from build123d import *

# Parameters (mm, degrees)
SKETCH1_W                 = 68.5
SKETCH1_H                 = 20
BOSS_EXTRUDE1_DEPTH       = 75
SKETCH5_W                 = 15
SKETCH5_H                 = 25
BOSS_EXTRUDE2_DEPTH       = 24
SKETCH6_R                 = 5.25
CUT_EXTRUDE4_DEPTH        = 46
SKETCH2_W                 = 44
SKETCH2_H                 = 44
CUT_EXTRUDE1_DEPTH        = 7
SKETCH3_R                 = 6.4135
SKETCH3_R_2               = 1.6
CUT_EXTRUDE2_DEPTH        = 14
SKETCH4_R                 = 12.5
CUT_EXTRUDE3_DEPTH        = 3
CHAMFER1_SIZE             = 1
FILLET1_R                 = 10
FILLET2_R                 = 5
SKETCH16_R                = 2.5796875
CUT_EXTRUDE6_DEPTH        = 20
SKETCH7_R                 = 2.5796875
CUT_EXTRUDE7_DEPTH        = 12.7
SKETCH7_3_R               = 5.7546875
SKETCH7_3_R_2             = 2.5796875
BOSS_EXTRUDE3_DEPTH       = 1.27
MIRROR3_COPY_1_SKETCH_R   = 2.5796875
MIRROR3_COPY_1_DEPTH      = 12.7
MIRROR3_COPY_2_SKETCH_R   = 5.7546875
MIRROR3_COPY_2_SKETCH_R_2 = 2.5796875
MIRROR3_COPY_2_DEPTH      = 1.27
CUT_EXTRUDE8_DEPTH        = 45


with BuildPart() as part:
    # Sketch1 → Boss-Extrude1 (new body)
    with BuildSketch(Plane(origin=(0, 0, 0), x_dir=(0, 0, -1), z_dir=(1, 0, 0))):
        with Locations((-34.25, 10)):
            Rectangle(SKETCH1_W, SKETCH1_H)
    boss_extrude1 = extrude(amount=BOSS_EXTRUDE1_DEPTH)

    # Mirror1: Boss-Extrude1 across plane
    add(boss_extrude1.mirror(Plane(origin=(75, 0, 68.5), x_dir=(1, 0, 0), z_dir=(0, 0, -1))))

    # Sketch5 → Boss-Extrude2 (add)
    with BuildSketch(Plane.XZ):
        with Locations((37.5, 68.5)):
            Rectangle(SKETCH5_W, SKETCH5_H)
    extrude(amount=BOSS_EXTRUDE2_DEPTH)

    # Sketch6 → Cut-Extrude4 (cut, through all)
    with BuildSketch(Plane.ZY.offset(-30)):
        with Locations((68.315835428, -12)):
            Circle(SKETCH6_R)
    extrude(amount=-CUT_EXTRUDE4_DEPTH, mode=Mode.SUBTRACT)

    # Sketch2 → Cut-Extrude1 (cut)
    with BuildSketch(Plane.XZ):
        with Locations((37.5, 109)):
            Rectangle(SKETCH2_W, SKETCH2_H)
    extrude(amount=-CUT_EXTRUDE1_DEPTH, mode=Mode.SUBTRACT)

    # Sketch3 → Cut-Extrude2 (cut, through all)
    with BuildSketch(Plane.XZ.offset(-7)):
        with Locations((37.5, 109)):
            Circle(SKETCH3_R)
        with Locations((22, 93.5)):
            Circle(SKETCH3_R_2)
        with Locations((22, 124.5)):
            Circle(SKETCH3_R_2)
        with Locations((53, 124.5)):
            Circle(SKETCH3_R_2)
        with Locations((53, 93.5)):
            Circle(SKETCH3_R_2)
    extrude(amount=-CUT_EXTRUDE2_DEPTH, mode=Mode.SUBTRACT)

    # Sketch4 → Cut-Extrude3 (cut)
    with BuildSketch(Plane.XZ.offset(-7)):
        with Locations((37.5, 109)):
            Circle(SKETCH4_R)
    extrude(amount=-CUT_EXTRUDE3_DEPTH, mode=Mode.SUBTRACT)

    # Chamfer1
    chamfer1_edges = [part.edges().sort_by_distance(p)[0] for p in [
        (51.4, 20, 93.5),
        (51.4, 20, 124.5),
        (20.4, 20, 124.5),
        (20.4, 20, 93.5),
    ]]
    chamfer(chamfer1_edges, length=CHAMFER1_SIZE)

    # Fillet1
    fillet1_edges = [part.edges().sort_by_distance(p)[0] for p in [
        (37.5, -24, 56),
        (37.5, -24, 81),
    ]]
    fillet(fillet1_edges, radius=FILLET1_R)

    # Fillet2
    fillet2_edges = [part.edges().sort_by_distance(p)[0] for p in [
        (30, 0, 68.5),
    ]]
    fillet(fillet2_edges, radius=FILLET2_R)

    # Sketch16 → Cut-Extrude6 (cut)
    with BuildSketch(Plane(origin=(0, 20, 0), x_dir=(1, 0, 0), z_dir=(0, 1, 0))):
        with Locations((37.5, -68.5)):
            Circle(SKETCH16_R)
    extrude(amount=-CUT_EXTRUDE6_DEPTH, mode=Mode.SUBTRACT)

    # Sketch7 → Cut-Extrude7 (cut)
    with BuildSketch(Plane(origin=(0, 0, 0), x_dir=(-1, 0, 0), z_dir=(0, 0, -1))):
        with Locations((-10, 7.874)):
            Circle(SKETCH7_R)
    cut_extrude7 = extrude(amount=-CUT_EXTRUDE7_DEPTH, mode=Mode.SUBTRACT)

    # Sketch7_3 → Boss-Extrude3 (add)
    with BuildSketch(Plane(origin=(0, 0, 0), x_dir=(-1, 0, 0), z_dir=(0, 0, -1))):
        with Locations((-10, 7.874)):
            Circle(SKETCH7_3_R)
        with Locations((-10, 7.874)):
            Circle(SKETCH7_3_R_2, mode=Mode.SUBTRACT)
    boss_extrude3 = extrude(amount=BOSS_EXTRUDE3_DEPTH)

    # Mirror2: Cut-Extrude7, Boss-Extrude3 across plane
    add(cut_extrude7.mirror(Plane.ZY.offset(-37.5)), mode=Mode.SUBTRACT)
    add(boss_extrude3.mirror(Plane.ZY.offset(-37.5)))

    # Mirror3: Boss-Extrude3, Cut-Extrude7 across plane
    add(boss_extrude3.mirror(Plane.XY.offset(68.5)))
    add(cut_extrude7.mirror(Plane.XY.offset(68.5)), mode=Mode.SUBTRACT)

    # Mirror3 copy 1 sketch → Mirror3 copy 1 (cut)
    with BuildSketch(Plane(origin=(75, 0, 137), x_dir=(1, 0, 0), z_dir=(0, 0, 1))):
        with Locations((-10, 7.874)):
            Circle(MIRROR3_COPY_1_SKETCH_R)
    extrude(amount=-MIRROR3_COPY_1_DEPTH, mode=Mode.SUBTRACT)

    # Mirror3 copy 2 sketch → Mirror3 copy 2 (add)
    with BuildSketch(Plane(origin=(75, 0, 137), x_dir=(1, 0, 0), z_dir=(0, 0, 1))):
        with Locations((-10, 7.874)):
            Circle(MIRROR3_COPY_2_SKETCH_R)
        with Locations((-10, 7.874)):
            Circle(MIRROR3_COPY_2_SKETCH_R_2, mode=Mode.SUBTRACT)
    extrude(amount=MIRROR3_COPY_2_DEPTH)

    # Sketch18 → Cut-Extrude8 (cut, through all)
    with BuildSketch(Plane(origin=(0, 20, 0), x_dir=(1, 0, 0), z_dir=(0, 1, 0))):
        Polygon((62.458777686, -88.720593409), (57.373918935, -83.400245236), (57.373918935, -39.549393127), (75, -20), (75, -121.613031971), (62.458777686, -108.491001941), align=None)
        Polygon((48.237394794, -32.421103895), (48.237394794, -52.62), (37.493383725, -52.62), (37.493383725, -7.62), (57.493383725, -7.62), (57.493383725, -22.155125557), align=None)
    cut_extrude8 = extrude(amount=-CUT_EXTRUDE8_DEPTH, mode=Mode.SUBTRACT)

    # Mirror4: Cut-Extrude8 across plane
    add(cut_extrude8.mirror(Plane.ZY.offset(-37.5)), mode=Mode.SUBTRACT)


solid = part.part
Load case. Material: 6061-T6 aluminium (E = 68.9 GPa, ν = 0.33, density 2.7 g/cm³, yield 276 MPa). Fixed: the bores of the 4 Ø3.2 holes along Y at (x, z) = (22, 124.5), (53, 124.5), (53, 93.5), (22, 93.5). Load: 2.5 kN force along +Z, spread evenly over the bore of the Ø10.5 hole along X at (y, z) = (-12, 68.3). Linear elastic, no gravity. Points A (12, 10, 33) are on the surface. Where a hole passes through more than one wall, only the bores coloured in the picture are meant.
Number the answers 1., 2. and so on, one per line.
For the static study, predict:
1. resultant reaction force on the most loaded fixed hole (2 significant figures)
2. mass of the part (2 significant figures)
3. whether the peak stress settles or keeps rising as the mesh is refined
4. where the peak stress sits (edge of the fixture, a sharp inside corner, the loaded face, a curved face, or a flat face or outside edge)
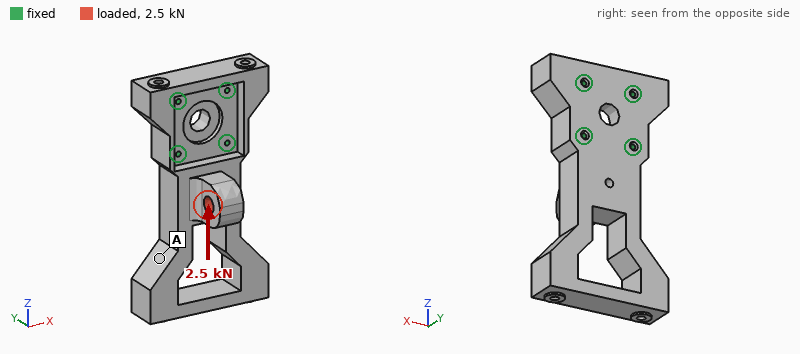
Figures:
1. 1.3 kN
2. 310 g
3. keeps rising
4. edge of the fixture
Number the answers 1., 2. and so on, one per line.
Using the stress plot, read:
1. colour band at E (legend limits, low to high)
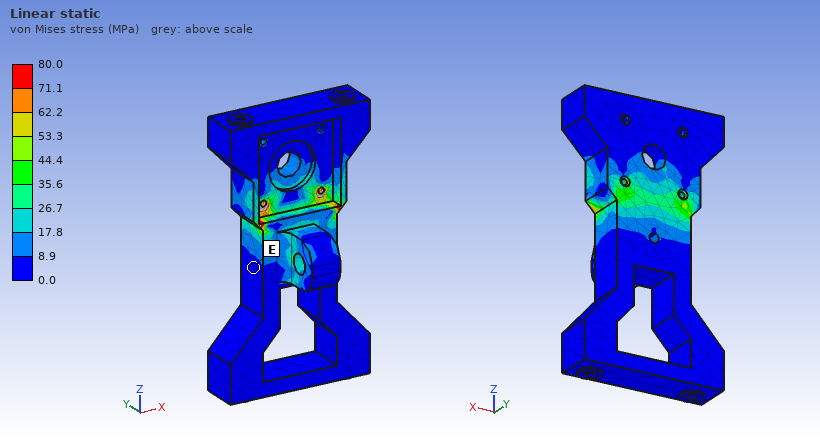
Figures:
1. 0.0 to 8.9 MPa
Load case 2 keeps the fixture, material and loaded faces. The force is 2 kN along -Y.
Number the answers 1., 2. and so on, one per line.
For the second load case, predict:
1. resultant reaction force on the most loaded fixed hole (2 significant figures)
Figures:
1. 1.3 kN
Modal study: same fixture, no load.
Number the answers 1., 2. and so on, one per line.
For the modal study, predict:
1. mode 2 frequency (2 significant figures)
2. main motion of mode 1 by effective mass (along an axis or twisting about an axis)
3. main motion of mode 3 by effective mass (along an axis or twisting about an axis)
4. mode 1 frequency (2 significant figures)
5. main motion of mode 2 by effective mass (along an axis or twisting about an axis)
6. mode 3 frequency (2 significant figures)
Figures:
1. 1500 Hz
2. along Y
3. twisting about Z
4. 1100 Hz
5. along X
6. 2500 Hz
